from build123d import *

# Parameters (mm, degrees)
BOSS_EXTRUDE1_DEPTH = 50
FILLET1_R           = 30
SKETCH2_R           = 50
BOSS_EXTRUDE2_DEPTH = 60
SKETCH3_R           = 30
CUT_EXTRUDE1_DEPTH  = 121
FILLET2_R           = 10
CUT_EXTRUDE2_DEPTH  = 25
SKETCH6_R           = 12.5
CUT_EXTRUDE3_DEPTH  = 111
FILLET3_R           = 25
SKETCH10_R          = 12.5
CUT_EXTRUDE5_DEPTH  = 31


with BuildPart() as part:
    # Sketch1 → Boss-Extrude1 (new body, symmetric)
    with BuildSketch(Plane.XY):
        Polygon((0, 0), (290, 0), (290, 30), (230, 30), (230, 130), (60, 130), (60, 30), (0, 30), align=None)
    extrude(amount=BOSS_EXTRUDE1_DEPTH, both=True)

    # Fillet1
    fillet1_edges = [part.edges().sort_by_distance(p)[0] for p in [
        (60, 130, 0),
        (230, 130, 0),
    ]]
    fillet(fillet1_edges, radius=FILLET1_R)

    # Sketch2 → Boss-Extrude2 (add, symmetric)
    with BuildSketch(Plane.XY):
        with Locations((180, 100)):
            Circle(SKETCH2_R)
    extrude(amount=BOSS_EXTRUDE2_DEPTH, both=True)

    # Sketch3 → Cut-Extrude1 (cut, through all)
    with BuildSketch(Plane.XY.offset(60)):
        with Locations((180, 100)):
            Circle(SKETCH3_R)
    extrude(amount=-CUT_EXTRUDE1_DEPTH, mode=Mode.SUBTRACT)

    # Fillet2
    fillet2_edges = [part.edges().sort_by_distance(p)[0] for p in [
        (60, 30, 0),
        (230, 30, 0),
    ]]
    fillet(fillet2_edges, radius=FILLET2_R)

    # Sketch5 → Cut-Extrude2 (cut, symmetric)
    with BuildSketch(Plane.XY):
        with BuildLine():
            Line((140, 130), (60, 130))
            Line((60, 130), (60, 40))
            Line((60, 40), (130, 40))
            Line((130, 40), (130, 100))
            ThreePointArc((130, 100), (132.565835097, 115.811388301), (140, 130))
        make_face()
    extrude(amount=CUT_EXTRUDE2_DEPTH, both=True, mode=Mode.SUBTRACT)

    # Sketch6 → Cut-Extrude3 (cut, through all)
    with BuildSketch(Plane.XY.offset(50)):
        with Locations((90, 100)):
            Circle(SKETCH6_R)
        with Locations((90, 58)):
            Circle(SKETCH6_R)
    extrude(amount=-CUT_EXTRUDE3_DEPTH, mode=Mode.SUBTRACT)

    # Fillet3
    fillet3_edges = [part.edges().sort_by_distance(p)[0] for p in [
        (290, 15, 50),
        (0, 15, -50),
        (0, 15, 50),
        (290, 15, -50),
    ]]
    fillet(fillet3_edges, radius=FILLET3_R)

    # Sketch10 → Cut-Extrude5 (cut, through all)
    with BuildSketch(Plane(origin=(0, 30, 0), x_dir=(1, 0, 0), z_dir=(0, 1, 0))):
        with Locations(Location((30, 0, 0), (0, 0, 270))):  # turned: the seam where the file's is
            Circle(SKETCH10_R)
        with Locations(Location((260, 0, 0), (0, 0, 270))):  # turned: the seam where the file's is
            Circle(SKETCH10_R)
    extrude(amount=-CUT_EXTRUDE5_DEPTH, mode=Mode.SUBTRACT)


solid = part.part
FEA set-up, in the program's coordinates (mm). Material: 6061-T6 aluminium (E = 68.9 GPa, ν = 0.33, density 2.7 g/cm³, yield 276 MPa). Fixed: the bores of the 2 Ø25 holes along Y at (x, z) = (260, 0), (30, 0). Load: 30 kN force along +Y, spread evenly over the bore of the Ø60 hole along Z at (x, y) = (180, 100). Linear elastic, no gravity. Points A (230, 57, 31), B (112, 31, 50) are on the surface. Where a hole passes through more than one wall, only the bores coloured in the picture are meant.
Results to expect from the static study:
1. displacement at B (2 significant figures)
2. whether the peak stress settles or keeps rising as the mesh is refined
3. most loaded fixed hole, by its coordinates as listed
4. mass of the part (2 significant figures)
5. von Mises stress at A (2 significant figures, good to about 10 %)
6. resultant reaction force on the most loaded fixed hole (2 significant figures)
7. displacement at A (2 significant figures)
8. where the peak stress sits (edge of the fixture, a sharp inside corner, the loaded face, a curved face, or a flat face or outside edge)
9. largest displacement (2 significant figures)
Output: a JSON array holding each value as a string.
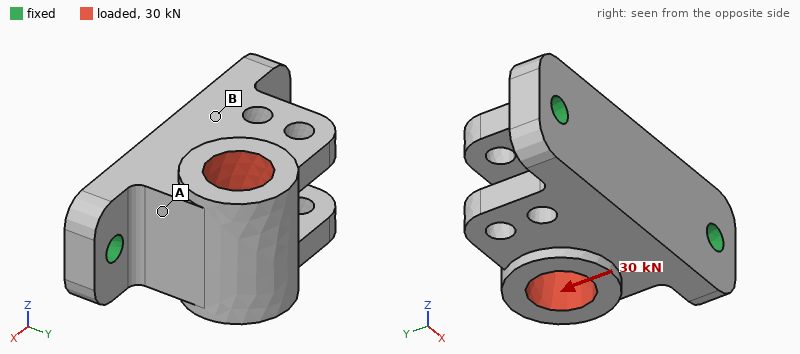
["23 µm", "keeps rising", "(260, 0)", "5.6 kg", "8.8 MPa", "22 kN", "23 µm", "edge of the fixture", "30 µm"]
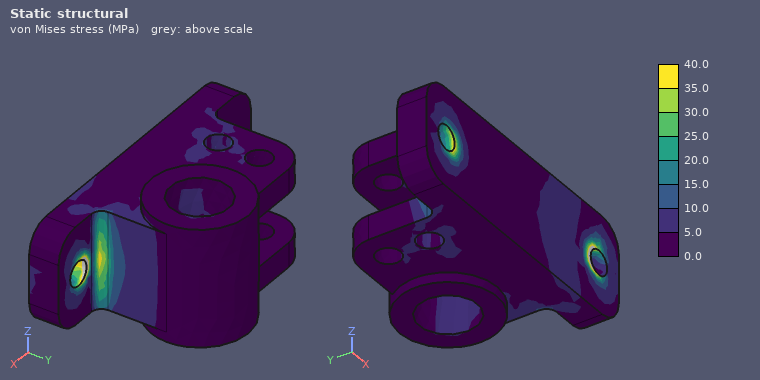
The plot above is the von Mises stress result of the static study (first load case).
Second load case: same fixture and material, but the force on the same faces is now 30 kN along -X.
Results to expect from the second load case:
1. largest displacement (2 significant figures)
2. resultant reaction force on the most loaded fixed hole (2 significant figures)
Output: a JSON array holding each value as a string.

["46 µm", "20 kN"]
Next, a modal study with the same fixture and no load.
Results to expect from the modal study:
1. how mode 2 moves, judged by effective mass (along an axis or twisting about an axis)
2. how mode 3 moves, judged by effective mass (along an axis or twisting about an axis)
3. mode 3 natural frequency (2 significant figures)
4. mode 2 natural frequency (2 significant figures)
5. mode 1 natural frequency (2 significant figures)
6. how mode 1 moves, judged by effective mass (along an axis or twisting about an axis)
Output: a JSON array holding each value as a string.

["along Y", "along X", "3000 Hz", "2500 Hz", "1100 Hz", "along Z"]
